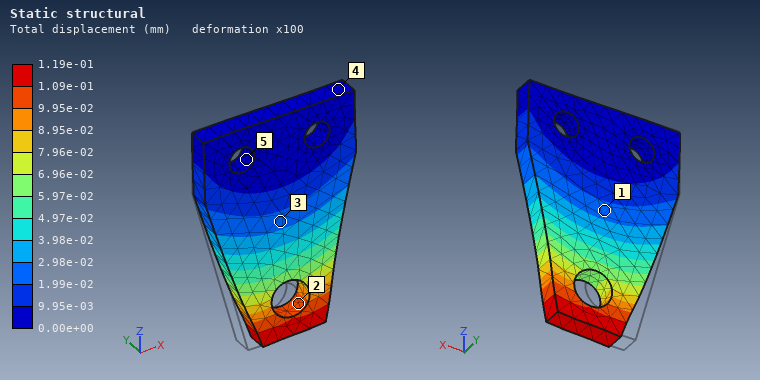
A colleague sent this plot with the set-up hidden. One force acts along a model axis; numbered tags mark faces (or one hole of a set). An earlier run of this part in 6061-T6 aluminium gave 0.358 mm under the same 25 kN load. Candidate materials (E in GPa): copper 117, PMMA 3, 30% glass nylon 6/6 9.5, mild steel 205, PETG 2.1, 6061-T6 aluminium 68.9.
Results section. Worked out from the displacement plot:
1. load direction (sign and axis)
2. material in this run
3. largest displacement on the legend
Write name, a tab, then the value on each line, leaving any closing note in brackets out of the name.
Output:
load direction	+X
material in this run	mild steel
largest displacement on the legend	1.19e-01 mm
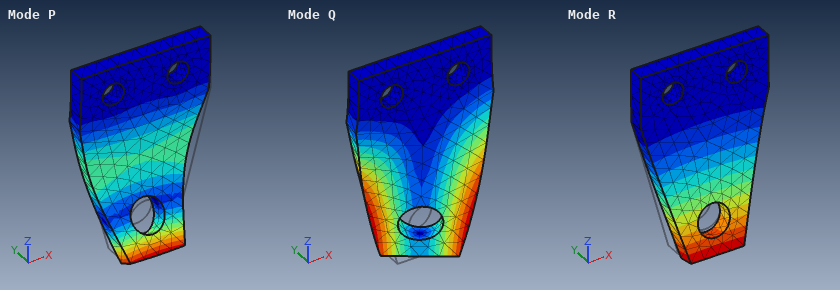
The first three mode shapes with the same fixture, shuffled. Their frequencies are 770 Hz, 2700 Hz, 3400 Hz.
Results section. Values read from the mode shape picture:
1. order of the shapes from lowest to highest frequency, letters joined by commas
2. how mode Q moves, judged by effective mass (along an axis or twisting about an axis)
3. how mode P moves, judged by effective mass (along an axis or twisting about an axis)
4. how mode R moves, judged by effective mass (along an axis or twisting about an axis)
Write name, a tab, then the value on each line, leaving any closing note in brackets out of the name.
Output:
order of the shapes from lowest to highest frequency, letters joined by commas	R, Q, P
how mode Q moves, judged by effective mass	twisting about Z
how mode P moves, judged by effective mass	along Y
how mode R moves, judged by effective mass	along Y
